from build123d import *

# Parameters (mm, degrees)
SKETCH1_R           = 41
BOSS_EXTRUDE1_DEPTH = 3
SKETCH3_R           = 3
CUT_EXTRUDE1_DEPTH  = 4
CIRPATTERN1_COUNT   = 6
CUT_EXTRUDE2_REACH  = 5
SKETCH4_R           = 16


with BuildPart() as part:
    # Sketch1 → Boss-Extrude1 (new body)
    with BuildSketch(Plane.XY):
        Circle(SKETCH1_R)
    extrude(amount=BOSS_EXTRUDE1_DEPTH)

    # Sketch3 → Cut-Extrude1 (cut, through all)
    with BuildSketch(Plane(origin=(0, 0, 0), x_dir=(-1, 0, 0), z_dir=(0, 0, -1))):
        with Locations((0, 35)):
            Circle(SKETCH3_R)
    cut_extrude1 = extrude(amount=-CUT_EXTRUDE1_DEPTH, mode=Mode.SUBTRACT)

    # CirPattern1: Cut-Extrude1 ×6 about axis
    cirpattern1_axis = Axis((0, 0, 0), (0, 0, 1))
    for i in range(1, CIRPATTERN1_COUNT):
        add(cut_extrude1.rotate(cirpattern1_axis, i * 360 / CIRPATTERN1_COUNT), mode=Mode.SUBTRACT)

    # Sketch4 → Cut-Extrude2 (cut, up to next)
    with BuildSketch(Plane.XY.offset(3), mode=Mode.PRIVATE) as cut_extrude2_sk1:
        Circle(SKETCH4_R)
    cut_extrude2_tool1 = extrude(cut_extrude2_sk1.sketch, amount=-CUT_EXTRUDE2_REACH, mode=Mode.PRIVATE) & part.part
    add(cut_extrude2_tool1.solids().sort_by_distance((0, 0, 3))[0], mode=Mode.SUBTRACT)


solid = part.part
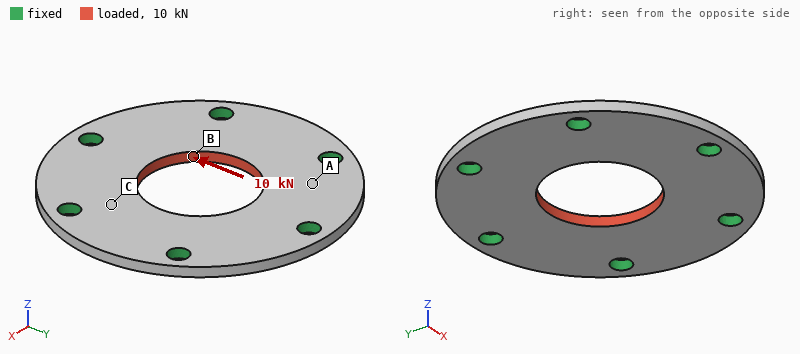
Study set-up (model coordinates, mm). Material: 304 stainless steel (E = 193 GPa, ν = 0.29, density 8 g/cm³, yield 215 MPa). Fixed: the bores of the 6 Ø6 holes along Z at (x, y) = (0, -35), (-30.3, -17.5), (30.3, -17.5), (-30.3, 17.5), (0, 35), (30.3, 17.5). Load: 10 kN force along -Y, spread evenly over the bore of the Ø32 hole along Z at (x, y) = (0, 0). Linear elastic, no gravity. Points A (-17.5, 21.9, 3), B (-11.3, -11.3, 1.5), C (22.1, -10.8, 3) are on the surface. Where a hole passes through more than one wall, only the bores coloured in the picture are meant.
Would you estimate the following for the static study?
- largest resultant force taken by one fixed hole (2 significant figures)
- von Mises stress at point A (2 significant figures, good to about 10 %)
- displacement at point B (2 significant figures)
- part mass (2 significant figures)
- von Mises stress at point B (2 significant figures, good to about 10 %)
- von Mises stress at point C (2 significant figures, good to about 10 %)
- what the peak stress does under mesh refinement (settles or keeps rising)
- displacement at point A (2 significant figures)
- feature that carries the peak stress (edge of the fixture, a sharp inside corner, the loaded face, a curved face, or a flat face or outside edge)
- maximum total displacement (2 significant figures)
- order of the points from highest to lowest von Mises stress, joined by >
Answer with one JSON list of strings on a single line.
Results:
["2.4 kN", "12 MPa", "4.7 µm", "100 g", "45 MPa", "31 MPa", "keeps rising", "2.7 µm", "edge of the fixture", "4.7 µm", "B > C > A"]
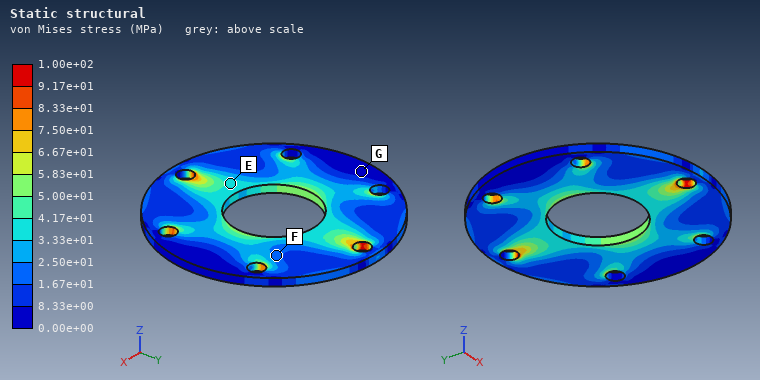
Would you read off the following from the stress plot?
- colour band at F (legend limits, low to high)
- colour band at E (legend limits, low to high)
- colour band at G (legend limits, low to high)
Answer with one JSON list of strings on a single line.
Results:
["1.67e+01 to 2.50e+01 MPa", "3.33e+01 to 4.17e+01 MPa", "0.00e+00 to 8.33e+00 MPa"]
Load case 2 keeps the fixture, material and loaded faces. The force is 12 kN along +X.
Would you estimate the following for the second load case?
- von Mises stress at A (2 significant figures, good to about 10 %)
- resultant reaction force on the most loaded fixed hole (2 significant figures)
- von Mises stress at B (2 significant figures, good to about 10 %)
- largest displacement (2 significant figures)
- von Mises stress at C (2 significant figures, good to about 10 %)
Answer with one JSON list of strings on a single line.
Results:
["27 MPa", "2.5 kN", "56 MPa", "5.6 µm", "50 MPa"]
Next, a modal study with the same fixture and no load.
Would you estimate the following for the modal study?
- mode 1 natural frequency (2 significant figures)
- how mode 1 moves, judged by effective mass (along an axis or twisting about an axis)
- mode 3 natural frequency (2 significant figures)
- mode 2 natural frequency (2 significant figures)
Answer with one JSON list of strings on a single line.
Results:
["8200 Hz", "along Z", "11 kHz", "11 kHz"]
